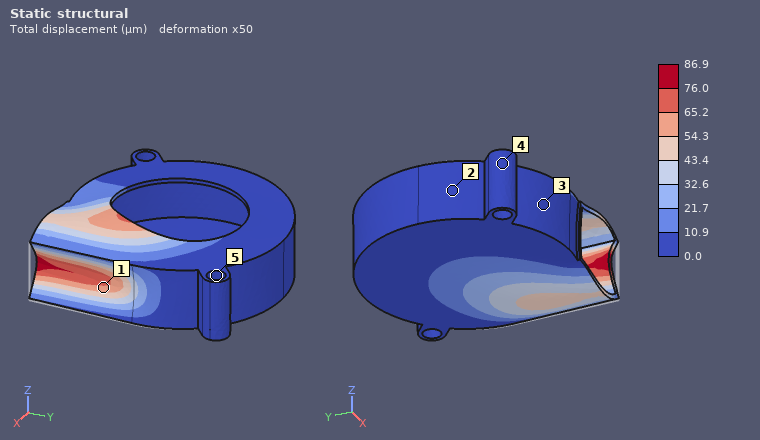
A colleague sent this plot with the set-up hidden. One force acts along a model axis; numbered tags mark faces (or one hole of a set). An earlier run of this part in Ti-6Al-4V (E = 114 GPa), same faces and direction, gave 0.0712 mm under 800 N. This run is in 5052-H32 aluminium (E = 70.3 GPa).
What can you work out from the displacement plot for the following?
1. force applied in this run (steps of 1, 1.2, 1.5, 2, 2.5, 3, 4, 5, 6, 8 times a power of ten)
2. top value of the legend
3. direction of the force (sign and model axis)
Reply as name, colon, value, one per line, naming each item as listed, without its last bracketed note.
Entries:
force applied in this run: 600 N
top value of the legend: 86.9 µm
direction of the force: -X
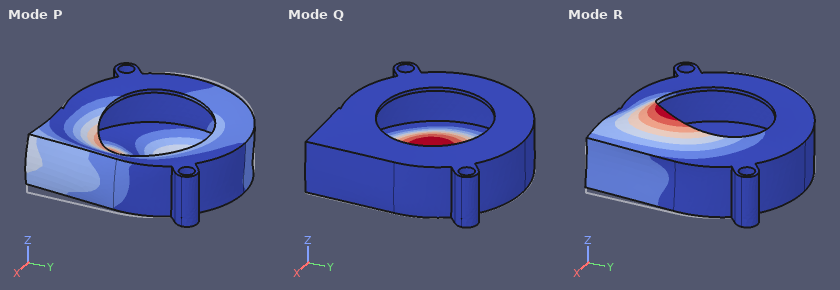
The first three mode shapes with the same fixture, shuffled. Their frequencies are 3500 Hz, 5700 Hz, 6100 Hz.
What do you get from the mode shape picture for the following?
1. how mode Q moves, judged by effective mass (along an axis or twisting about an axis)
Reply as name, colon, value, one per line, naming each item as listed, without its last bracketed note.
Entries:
how mode Q moves, judged by effective mass: along Z
